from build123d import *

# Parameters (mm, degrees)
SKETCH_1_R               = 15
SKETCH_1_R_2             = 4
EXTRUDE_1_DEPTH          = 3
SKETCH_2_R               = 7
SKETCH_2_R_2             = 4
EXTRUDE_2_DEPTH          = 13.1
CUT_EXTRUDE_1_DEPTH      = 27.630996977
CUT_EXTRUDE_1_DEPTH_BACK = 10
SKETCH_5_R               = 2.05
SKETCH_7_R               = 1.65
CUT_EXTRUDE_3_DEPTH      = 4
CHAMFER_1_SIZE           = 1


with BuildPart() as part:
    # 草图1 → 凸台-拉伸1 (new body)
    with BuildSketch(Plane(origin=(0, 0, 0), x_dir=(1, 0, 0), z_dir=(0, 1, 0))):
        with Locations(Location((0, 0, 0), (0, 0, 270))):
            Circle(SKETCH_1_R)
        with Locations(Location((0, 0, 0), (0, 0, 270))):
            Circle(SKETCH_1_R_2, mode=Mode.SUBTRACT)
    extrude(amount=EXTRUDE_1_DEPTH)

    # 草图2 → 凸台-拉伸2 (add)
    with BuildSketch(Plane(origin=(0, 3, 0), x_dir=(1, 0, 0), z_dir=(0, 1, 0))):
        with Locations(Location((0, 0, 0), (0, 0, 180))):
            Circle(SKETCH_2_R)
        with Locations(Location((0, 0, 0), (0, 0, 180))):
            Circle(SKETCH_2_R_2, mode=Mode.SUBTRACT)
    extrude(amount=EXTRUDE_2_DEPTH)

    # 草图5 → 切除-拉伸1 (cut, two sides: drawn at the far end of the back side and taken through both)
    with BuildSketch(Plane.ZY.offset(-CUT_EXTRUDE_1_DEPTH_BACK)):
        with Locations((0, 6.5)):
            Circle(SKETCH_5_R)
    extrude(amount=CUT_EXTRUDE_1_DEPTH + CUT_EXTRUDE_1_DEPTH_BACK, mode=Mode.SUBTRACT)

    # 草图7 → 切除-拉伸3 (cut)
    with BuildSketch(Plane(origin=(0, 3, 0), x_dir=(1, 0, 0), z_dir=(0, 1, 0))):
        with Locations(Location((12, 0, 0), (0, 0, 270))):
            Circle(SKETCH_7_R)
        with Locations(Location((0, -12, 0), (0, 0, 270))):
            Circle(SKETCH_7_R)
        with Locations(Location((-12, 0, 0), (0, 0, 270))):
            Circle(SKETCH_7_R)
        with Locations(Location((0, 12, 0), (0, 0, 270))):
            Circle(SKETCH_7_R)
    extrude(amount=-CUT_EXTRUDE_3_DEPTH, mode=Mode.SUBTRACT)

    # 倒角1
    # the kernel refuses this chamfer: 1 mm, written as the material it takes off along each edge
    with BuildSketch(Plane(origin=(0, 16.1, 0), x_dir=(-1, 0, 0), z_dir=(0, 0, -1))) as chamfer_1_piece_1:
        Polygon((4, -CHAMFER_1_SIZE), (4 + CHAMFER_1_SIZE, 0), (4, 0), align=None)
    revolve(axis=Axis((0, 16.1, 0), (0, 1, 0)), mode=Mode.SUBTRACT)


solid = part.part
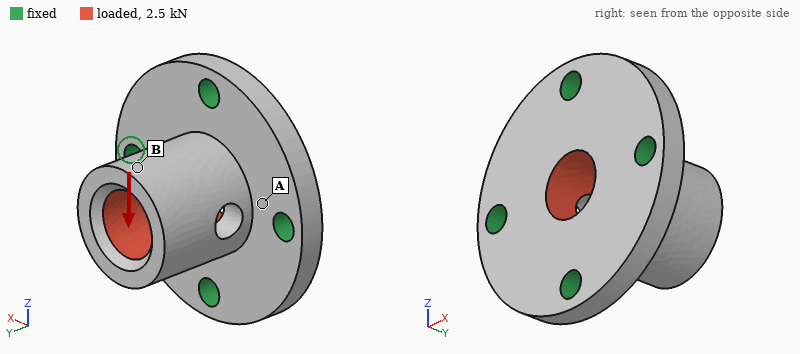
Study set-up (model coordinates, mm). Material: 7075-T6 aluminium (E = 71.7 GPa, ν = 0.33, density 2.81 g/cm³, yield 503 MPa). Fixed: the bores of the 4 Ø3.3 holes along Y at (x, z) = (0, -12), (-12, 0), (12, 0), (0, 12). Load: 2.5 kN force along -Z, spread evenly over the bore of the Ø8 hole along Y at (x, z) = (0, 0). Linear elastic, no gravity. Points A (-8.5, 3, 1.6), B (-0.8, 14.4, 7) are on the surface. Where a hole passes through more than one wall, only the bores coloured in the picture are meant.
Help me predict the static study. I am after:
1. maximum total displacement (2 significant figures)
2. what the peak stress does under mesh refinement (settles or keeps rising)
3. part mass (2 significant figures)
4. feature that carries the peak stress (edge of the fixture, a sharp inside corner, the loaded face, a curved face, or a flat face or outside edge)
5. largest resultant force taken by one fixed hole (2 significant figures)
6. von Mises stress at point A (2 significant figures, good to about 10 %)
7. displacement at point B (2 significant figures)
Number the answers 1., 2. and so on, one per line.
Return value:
1. 40 µm
2. keeps rising
3. 8.8 g
4. edge of the fixture
5. 1.1 kN
6. 38 MPa
7. 37 µm
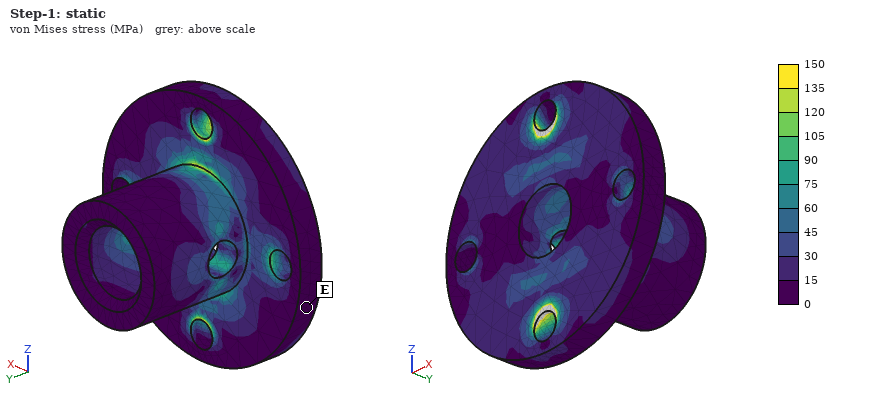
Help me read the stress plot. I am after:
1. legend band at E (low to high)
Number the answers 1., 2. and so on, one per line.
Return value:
1. 0 to 15 MPa
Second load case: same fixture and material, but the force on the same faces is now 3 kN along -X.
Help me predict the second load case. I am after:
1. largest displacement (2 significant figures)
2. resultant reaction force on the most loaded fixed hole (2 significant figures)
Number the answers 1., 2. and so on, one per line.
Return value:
1. 50 µm
2. 1.3 kN
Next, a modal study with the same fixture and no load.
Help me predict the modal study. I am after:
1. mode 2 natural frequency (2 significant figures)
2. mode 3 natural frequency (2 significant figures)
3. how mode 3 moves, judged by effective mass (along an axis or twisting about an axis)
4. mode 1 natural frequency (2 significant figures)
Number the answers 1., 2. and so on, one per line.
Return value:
1. 21 kHz
2. 31 kHz
3. along Y
4. 20 kHz
